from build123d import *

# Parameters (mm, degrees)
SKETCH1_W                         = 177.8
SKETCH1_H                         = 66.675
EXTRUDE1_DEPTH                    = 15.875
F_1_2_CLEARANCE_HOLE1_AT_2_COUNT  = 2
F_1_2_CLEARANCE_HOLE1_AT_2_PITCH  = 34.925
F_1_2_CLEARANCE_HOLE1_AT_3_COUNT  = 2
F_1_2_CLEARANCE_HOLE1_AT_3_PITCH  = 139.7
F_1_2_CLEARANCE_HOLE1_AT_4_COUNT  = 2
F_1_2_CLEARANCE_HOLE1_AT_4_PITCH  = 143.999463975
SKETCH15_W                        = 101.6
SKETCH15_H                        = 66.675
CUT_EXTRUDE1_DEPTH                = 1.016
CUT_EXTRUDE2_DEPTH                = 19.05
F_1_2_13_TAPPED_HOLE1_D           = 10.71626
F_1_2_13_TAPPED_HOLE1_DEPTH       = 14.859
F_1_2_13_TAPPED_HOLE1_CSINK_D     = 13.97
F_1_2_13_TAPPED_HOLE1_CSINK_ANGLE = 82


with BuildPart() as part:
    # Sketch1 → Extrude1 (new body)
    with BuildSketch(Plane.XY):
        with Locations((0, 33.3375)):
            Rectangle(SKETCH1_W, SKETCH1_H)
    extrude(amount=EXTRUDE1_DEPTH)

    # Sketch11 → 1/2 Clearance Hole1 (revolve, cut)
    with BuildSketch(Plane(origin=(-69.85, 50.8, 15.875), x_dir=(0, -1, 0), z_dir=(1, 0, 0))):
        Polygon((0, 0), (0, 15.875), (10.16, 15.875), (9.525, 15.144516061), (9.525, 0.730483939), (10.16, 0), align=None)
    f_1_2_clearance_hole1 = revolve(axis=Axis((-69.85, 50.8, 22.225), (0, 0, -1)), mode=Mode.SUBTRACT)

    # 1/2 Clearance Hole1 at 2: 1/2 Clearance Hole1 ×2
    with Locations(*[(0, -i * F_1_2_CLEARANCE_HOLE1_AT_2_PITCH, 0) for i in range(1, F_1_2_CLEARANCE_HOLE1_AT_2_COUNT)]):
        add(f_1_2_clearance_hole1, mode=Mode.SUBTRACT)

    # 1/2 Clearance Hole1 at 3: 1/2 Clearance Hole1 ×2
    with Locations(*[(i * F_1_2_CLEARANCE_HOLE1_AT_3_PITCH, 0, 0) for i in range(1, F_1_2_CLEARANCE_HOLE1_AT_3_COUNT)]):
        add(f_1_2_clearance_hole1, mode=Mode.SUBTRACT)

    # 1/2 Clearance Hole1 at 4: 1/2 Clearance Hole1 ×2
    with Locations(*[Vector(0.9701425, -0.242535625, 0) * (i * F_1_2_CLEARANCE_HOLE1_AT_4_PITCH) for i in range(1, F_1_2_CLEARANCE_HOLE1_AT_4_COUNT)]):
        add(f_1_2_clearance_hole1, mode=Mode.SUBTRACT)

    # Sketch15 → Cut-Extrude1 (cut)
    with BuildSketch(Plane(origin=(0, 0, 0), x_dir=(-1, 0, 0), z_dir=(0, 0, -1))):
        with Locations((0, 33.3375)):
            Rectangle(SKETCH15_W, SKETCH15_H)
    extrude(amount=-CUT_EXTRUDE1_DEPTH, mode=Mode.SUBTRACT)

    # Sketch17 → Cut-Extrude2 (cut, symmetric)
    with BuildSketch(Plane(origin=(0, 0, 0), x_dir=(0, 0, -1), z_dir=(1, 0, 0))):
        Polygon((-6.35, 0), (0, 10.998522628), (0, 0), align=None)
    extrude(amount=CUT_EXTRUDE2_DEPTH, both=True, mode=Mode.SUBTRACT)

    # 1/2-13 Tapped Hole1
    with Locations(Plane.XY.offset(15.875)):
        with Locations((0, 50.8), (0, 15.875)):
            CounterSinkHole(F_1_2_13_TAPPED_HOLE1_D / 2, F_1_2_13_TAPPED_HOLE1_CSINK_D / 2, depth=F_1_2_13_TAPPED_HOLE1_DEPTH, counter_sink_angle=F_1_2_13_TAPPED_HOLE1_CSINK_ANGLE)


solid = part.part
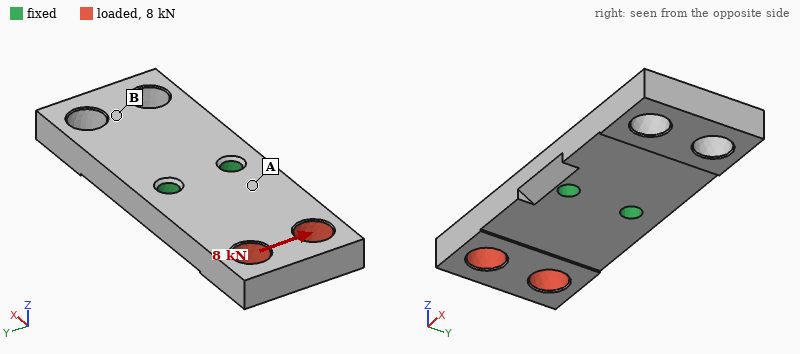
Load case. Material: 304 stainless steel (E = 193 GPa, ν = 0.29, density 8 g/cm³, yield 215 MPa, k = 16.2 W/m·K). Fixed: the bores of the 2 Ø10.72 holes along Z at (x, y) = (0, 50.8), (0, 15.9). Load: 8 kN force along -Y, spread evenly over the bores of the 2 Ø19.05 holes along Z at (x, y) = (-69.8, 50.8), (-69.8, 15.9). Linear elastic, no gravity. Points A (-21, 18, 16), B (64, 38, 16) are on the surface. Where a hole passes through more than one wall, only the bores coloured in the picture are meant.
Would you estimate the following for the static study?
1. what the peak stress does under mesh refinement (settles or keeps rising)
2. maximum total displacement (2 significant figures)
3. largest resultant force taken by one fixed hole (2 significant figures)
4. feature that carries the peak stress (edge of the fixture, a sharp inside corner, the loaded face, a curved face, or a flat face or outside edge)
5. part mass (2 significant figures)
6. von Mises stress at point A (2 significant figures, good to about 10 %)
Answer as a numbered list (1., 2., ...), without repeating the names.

1. keeps rising
2. 36 µm
3. 14 kN
4. edge of the fixture
5. 1.3 kg
6. 26 MPa
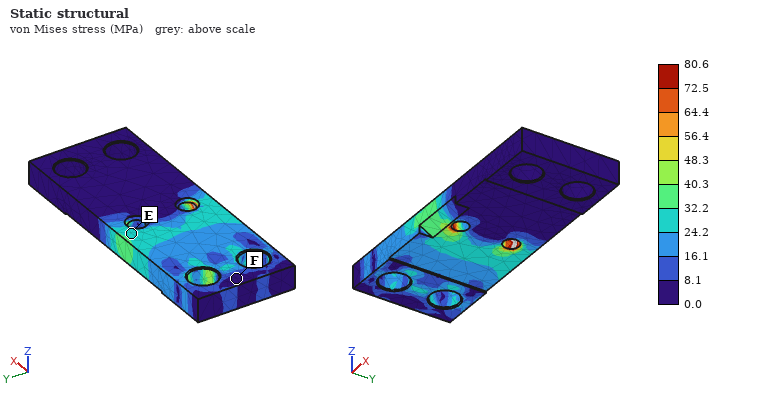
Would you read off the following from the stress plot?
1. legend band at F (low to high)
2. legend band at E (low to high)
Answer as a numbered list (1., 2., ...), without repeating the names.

1. 0.0 to 8.1 MPa
2. 24.2 to 32.2 MPa
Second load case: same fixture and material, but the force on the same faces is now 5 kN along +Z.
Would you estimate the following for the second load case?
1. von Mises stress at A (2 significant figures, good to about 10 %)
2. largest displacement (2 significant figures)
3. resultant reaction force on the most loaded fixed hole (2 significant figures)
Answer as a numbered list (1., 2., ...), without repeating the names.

1. 96 MPa
2. 0.24 mm
3. 2.5 kN
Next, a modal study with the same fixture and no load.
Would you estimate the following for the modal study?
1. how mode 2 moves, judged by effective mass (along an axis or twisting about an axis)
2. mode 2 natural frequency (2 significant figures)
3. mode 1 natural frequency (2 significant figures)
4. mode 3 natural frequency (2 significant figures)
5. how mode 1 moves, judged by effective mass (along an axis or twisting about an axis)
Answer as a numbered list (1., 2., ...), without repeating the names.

1. along Z
2. 1600 Hz
3. 1500 Hz
4. 4100 Hz
5. twisting about Y
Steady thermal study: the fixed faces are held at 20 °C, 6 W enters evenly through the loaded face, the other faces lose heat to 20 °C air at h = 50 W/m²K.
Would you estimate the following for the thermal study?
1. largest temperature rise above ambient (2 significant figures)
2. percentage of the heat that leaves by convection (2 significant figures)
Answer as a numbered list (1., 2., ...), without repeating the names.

1. 12 K
2. 72 %
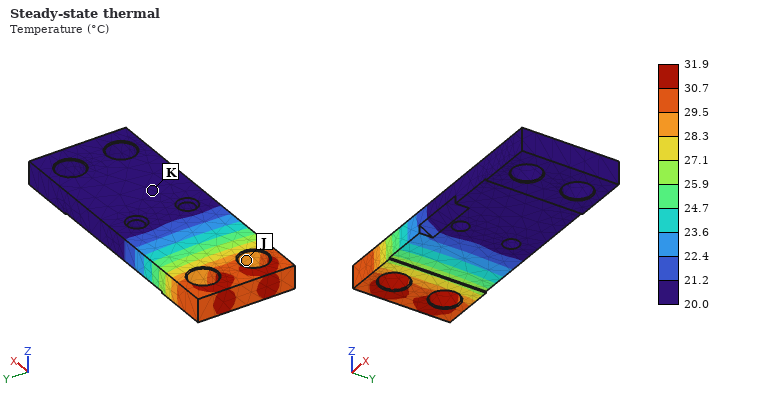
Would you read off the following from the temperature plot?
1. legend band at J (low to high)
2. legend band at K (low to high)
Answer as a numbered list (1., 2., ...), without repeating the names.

1. 28.3 to 29.5 °C
2. 20.0 to 21.2 °C
